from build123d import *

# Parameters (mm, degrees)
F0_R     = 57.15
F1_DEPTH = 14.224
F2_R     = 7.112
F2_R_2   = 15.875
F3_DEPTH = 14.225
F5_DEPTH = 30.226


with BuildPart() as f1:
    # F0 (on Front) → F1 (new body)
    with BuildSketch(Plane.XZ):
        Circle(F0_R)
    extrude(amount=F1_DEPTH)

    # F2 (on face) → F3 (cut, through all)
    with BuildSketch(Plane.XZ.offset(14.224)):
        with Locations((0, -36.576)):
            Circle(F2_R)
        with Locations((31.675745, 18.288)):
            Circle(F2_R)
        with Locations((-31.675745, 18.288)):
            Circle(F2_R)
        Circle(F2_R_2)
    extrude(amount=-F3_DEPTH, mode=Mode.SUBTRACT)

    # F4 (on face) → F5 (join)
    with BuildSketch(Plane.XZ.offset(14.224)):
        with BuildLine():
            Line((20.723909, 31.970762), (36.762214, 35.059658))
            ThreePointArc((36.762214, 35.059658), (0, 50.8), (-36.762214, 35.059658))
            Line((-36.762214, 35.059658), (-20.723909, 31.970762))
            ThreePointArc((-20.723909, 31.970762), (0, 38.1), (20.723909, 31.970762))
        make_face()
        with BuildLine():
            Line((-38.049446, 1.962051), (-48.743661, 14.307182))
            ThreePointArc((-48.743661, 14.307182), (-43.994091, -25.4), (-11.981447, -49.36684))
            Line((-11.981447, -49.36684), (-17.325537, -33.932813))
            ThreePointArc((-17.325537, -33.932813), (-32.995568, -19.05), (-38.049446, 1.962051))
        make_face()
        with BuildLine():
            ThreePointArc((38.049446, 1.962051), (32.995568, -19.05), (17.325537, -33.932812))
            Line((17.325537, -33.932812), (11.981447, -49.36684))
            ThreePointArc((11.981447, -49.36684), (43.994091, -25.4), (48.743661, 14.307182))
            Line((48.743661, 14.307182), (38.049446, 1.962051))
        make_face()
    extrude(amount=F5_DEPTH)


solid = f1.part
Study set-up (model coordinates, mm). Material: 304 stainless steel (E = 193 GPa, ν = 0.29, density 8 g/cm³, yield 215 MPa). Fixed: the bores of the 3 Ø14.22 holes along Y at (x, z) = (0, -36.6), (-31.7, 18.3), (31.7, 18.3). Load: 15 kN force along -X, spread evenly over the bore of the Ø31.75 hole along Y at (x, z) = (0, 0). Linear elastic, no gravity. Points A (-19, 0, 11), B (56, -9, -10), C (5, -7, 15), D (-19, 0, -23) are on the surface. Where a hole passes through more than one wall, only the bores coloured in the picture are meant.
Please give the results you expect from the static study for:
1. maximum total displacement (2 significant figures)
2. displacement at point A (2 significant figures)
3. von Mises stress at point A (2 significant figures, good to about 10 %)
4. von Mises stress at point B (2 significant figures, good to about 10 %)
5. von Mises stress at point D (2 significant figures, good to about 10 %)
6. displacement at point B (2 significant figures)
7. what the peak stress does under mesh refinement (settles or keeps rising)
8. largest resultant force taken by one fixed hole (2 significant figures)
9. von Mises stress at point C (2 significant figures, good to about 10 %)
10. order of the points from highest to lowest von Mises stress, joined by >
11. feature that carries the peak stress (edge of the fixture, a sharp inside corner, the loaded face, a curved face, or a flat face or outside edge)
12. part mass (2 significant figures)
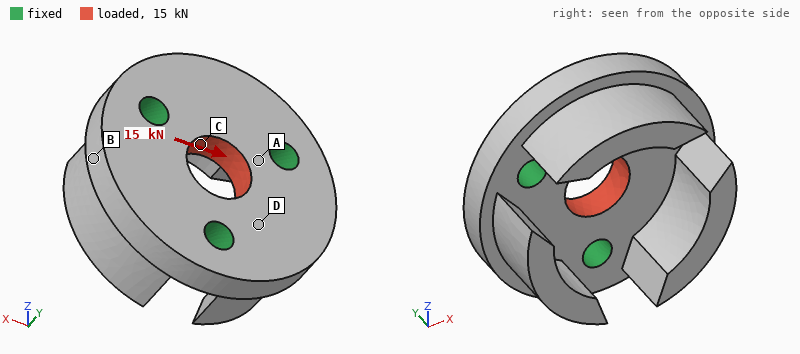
2.1 µm
0.72 µm
13 MPa
3.6 MPa
6.9 MPa
0.88 µm
keeps rising
5.2 kN
17 MPa
C > A > D > B
edge of the fixture
1.6 kg
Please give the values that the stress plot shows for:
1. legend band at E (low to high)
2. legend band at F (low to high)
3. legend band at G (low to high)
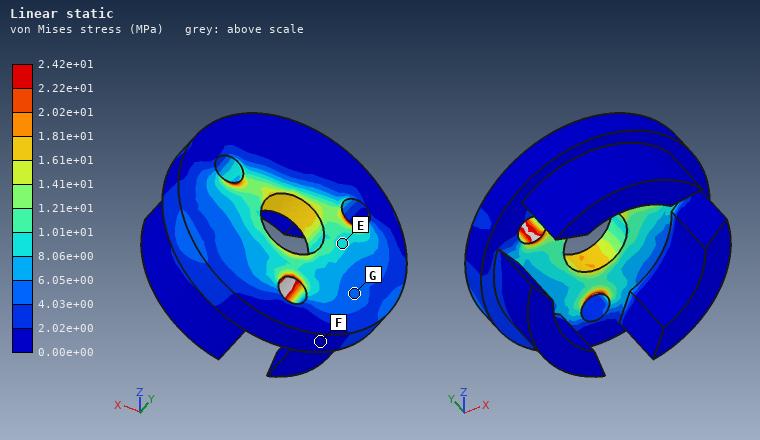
8.06e+00 to 1.01e+01 MPa
0.00e+00 to 2.02e+00 MPa
4.03e+00 to 6.05e+00 MPa
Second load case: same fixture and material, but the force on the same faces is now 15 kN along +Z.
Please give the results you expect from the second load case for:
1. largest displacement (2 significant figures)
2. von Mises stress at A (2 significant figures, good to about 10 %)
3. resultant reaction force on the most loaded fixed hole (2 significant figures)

2.3 µm
11 MPa
5.1 kN
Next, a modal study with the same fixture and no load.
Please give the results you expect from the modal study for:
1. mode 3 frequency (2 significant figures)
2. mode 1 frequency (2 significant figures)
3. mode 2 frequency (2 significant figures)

4400 Hz
4300 Hz
4300 Hz
